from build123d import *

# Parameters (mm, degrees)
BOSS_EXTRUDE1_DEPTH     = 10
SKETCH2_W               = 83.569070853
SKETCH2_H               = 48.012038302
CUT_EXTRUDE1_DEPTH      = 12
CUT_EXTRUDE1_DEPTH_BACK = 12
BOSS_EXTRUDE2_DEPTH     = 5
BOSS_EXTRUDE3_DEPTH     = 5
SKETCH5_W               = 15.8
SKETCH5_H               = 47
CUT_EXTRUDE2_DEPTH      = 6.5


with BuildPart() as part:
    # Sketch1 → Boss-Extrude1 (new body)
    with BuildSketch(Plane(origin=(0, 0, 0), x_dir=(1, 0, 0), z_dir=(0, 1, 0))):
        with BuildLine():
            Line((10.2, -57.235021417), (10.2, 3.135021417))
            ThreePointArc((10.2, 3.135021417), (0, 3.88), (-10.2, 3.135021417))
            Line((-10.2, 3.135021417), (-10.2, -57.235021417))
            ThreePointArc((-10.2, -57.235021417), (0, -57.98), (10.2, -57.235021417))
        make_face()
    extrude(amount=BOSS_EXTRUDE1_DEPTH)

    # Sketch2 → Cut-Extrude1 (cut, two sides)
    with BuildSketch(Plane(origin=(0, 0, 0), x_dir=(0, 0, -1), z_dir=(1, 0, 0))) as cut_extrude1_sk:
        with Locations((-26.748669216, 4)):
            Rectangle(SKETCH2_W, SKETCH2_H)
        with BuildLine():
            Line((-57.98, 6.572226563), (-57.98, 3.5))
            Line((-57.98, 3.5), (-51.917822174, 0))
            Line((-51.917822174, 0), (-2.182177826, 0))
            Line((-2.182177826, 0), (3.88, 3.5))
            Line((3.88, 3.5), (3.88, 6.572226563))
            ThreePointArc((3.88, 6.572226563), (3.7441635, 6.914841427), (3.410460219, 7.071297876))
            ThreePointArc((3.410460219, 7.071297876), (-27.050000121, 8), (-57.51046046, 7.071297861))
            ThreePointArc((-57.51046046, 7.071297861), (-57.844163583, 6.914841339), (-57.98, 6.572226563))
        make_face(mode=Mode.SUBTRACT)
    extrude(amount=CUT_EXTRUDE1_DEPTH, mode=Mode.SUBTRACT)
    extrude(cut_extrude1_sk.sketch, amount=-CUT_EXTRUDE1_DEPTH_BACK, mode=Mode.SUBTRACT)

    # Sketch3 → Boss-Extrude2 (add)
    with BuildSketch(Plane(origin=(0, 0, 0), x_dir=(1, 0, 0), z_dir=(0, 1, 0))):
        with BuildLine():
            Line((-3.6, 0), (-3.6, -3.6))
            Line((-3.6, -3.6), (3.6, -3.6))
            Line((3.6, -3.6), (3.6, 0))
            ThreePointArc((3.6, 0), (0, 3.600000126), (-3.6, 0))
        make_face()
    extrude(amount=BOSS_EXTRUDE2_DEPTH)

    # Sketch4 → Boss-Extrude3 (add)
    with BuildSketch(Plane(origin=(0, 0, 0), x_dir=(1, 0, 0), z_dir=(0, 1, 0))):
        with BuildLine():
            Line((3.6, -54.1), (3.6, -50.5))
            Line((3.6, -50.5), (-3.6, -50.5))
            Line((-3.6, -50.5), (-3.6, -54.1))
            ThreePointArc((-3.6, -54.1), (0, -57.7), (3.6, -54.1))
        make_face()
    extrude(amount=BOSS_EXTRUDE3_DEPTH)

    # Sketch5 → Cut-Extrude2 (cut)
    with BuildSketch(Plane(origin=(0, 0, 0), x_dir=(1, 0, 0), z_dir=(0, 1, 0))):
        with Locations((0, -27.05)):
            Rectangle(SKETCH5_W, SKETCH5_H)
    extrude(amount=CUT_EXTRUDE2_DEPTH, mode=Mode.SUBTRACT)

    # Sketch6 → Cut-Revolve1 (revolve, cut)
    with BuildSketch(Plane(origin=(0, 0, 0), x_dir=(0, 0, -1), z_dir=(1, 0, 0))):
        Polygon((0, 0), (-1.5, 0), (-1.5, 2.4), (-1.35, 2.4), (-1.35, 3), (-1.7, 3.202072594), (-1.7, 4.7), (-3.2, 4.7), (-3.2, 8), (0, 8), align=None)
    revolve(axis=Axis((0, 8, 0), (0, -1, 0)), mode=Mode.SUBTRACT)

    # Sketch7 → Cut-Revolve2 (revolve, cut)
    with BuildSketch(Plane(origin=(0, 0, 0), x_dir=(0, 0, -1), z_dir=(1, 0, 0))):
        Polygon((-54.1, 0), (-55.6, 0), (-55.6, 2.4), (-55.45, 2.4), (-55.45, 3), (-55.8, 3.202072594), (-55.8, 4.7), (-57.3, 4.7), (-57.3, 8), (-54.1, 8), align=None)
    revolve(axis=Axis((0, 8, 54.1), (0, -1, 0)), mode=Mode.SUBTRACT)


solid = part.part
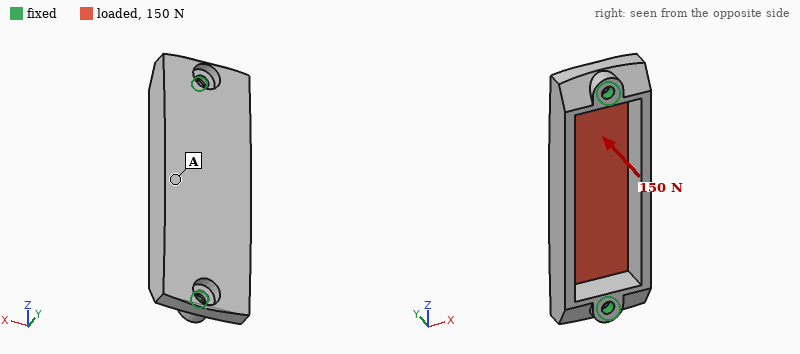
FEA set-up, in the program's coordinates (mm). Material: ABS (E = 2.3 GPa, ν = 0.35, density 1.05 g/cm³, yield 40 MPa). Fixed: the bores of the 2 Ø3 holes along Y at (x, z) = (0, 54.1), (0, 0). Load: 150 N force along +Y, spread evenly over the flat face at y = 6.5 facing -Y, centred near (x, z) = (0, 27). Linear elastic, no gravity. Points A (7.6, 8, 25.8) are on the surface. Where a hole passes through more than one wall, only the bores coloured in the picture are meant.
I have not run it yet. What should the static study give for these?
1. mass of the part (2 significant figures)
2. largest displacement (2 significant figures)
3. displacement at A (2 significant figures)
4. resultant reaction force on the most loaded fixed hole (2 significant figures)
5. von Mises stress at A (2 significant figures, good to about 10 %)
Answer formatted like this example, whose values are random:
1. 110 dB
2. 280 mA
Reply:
1. 4.5 g
2. 0.48 mm
3. 0.33 mm
4. 90 N
5. 6.6 MPa
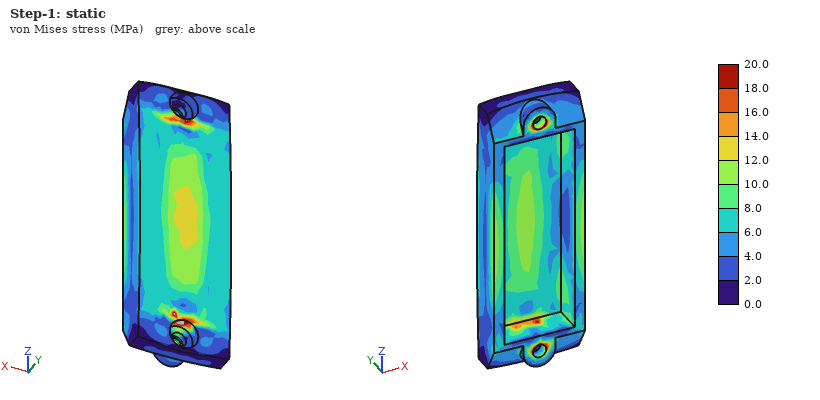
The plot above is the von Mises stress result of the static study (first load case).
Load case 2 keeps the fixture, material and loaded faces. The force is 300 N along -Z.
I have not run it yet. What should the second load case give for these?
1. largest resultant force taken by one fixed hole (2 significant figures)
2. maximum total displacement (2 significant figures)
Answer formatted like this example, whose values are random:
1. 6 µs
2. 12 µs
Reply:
1. 150 N
2. 86 µm
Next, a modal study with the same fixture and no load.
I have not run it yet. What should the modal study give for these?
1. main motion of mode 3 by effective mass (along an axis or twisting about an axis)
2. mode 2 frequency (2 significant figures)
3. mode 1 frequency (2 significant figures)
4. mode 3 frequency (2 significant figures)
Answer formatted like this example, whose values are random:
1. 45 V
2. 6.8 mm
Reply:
1. along X
2. 2200 Hz
3. 2200 Hz
4. 3000 Hz
